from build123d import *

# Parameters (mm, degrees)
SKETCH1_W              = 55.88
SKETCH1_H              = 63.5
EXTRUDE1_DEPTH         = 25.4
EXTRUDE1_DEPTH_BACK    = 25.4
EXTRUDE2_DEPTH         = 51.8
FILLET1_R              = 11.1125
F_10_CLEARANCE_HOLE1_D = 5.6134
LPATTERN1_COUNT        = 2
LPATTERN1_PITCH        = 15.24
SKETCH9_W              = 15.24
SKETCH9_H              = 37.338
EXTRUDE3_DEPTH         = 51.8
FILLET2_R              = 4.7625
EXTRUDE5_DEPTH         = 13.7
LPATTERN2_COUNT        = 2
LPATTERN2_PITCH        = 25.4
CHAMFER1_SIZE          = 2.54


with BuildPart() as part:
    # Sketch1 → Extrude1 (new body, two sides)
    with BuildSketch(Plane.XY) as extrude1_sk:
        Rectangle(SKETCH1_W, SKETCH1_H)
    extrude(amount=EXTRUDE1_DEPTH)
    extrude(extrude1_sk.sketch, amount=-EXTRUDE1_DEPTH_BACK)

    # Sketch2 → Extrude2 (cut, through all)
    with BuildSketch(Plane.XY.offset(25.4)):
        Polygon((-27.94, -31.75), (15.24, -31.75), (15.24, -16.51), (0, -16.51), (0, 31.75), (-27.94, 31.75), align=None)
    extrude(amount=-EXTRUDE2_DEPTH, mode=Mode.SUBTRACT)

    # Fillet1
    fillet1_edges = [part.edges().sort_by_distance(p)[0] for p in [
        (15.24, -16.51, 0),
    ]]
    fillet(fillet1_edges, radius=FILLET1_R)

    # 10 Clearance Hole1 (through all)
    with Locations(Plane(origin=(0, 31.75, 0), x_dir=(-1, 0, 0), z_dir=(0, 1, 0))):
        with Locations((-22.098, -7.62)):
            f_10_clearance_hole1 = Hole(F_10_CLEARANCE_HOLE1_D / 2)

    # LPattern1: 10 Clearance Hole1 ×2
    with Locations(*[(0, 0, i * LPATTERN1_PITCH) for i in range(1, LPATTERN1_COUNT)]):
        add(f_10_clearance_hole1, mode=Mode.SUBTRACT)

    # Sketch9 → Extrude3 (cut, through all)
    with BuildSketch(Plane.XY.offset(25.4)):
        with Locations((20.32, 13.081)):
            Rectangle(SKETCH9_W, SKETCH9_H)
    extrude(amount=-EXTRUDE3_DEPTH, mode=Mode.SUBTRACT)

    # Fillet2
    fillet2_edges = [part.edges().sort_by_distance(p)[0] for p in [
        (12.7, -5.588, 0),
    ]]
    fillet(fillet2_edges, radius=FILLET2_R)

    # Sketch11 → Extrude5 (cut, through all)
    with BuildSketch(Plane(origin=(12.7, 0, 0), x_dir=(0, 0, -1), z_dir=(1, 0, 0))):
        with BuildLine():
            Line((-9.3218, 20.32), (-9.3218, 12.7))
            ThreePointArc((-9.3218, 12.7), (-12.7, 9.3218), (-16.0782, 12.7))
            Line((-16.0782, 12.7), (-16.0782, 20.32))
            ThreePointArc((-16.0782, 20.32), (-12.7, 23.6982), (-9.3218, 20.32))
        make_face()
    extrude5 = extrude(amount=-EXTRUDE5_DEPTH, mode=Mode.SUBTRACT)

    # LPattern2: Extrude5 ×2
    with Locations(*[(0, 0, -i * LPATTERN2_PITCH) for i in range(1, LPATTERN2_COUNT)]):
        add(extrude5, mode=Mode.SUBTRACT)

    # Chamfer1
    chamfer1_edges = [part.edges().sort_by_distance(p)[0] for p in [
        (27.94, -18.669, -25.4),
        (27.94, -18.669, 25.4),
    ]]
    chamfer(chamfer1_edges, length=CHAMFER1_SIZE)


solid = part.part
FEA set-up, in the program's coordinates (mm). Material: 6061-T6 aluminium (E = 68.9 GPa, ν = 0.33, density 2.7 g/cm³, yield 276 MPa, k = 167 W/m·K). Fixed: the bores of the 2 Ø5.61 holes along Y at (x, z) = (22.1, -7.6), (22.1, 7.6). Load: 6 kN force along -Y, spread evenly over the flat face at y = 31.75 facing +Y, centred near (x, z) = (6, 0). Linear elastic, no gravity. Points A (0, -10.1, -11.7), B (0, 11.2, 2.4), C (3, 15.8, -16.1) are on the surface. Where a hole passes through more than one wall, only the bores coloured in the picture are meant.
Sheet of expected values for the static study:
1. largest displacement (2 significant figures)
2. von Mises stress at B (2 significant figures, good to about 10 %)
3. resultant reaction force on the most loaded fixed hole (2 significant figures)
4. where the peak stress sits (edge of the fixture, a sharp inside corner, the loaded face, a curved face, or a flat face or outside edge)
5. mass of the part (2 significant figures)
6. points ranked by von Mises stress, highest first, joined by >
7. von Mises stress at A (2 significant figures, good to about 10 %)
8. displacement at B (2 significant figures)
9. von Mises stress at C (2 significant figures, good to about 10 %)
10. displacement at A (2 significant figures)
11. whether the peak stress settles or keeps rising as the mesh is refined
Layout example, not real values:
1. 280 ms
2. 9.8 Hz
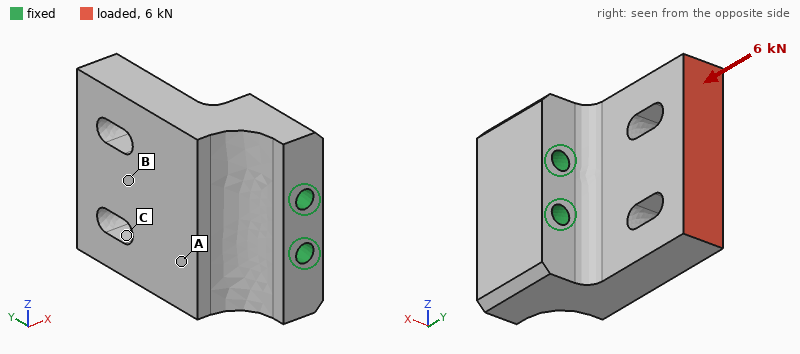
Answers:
1. 43 µm
2. 12 MPa
3. 3.0 kN
4. edge of the fixture
5. 130 g
6. C > B > A
7. 5.1 MPa
8. 27 µm
9. 17 MPa
10. 16 µm
11. keeps rising
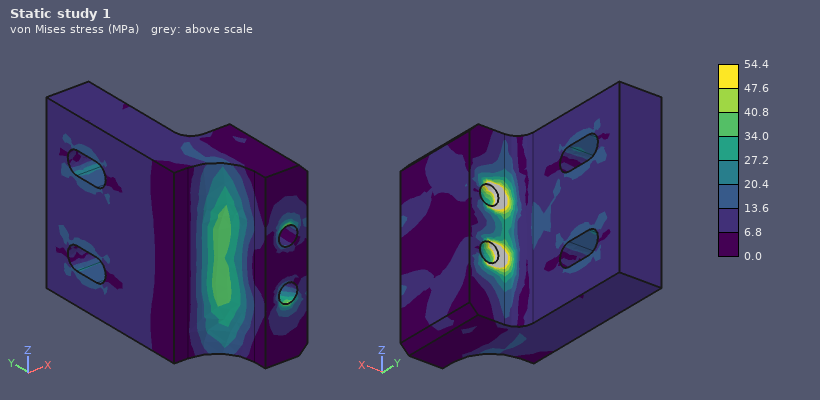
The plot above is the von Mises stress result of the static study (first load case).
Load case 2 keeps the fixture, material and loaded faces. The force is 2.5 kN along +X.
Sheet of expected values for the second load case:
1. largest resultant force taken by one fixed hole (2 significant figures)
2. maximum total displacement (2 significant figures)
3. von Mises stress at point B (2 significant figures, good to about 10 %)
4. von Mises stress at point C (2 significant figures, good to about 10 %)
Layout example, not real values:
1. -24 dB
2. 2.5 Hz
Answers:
1. 1.3 kN
2. 0.17 mm
3. 43 MPa
4. 26 MPa
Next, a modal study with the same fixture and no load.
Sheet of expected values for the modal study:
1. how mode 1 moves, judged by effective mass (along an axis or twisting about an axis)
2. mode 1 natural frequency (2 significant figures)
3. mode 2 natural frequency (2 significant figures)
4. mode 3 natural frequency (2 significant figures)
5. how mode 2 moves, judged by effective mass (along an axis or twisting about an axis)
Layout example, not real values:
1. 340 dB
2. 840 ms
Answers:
1. along X
2. 4500 Hz
3. 7100 Hz
4. 8600 Hz
5. along Z
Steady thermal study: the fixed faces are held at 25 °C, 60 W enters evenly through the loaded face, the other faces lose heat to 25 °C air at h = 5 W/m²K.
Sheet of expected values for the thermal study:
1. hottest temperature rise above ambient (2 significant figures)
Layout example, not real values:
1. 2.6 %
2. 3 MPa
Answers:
1. 32 K
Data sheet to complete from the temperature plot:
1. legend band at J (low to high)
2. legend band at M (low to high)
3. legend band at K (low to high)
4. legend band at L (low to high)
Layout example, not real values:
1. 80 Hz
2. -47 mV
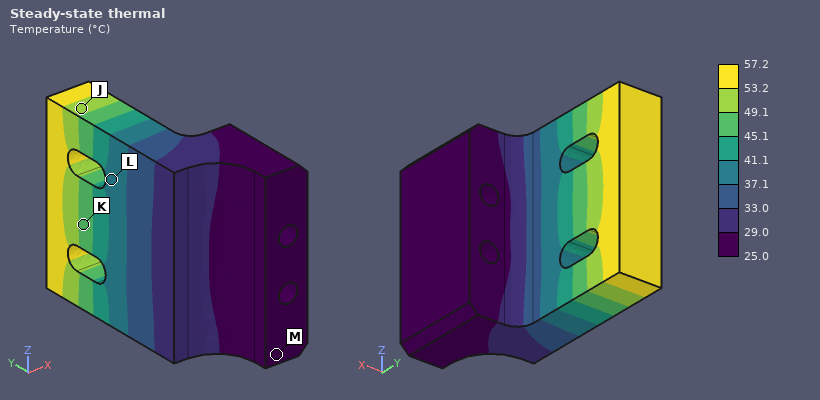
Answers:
1. 49.1 to 53.2 °C
2. 25.0 to 29.0 °C
3. 45.1 to 49.1 °C
4. 37.1 to 41.1 °C
